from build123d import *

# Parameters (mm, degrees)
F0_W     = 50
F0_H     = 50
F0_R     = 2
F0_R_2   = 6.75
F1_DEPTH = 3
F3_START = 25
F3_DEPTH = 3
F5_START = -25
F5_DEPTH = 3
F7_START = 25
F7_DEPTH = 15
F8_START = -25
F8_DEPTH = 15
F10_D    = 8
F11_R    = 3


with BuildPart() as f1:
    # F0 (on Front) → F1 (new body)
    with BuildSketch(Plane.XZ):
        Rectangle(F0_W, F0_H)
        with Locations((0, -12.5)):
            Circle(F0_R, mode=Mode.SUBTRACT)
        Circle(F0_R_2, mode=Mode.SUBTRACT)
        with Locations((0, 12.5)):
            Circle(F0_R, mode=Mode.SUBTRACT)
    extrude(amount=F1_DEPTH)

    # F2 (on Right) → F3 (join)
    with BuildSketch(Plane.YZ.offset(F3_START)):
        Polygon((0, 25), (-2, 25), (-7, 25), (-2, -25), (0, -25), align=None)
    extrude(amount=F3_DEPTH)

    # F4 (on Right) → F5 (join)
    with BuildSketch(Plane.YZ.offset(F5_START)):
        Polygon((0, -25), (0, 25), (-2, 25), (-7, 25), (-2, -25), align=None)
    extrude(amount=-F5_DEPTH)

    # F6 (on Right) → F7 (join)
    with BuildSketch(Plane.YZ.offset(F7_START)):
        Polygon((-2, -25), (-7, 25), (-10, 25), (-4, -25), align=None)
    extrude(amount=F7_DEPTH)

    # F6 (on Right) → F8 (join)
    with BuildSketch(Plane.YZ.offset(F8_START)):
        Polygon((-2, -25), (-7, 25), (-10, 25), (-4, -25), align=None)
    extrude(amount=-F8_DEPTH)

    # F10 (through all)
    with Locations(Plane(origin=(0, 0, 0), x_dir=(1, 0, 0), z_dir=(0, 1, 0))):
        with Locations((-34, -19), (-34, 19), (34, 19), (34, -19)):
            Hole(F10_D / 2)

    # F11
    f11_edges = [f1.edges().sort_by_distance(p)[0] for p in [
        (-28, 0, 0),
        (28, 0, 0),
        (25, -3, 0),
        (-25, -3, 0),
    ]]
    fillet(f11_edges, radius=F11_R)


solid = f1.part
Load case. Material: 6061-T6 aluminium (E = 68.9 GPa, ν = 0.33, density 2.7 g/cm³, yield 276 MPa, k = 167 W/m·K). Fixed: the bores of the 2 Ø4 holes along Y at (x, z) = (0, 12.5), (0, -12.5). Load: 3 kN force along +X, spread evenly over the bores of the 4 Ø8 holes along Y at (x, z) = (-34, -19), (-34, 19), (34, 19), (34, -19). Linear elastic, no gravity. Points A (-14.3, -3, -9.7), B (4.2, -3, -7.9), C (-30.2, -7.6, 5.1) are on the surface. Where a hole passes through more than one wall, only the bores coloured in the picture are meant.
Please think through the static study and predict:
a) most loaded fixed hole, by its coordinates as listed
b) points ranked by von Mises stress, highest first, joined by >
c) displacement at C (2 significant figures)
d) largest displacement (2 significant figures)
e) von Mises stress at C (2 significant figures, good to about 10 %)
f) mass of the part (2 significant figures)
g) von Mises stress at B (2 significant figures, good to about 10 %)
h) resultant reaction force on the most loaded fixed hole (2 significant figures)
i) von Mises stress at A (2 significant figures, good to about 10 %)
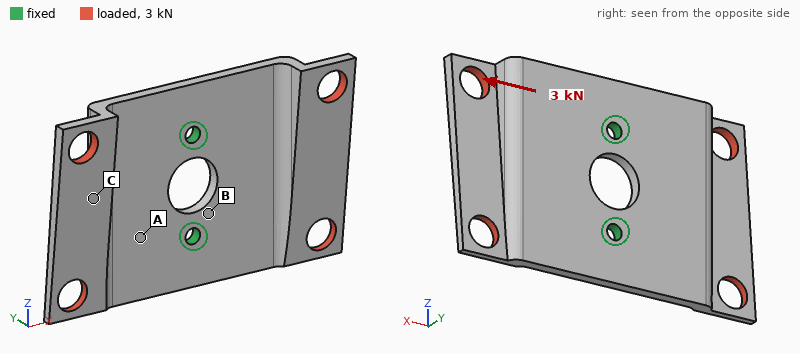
(0, 12.5)
B > A > C
0.48 mm
0.84 mm
34 MPa
31 g
140 MPa
1.8 kN
83 MPa
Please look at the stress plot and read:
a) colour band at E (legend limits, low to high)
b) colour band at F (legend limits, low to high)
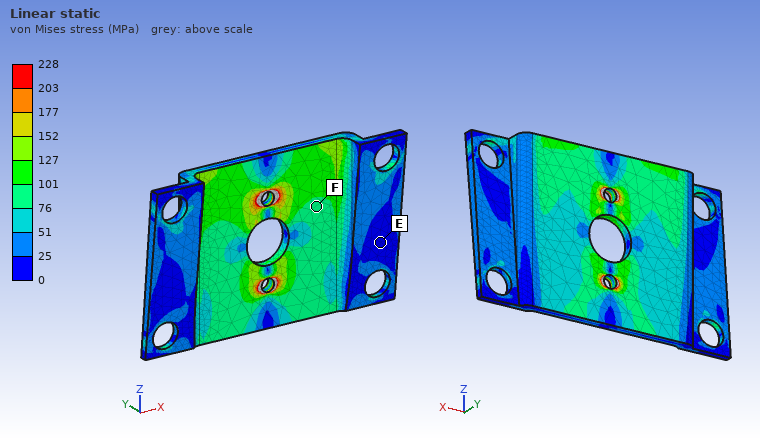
0 to 25 MPa
76 to 101 MPa
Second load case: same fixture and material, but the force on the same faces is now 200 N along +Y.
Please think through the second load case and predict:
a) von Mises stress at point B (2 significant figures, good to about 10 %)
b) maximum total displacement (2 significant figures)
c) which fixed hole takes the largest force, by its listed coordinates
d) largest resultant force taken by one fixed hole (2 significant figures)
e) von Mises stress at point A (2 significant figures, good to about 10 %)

50 MPa
0.25 mm
(0, 12.5)
120 N
23 MPa
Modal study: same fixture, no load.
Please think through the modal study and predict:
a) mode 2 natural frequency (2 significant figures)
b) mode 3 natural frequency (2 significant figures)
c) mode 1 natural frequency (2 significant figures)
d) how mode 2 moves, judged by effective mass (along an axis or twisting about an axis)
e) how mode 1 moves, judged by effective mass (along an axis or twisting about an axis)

1600 Hz
3200 Hz
1500 Hz
along Y
twisting about Z
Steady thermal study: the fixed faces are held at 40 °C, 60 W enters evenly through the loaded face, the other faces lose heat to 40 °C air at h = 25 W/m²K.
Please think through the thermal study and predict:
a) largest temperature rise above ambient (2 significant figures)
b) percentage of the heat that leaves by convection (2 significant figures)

70 K
11 %
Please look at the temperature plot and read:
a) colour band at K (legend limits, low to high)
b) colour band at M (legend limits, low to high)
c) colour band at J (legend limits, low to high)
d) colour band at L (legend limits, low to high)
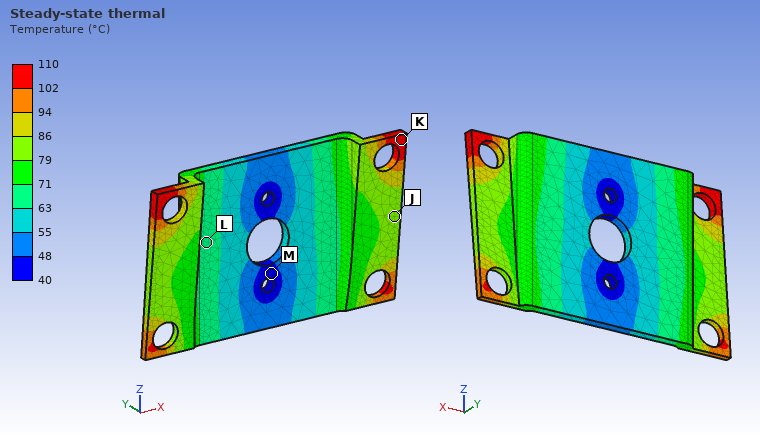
102 to 110 °C
40 to 48 °C
79 to 86 °C
63 to 71 °C
